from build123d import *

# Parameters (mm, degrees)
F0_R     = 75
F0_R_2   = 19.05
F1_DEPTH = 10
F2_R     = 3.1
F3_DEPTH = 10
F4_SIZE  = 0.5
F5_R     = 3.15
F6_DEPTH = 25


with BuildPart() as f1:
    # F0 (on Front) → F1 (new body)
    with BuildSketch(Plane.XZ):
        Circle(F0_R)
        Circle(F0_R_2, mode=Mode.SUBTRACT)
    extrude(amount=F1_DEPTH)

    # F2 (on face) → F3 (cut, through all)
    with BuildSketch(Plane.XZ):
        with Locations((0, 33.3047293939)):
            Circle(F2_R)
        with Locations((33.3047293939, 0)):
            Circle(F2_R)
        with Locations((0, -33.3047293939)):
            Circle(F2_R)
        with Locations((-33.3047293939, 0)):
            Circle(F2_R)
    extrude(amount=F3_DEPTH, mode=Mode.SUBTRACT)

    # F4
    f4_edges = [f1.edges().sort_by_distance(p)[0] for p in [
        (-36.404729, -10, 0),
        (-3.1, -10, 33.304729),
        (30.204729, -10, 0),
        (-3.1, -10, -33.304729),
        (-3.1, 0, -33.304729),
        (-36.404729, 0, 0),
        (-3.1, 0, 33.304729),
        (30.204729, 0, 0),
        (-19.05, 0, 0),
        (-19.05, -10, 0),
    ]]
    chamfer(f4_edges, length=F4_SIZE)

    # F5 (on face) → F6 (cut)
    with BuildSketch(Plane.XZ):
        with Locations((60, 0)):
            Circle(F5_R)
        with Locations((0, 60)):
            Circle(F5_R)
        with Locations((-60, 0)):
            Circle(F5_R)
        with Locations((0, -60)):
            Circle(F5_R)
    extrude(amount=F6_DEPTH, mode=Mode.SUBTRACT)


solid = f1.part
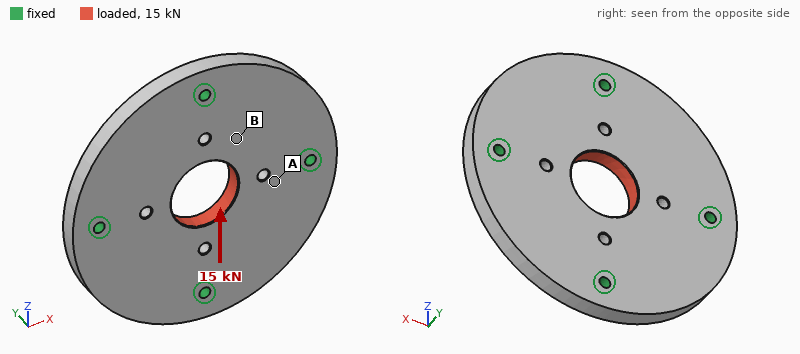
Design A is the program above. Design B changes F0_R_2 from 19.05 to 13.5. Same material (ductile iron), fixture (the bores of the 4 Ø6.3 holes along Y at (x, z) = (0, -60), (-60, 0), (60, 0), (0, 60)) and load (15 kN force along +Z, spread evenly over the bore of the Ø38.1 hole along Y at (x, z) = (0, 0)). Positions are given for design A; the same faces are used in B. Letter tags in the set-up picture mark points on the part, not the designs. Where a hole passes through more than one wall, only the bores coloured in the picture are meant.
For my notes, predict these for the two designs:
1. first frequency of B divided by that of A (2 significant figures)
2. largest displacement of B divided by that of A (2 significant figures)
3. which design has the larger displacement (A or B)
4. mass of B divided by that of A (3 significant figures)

1.0
1.2
B
1.03
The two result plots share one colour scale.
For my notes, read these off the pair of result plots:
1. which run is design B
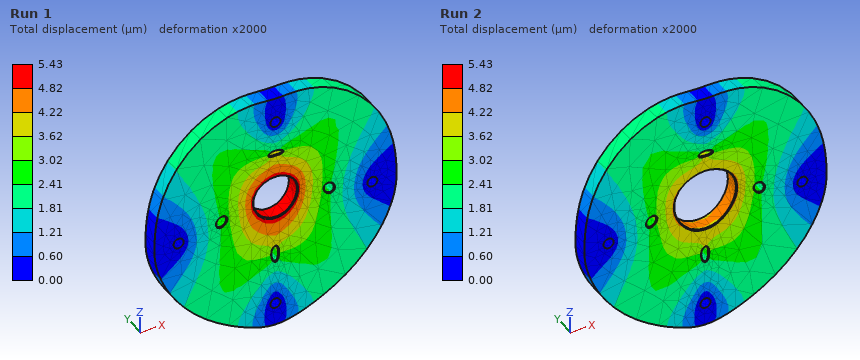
Run 1
